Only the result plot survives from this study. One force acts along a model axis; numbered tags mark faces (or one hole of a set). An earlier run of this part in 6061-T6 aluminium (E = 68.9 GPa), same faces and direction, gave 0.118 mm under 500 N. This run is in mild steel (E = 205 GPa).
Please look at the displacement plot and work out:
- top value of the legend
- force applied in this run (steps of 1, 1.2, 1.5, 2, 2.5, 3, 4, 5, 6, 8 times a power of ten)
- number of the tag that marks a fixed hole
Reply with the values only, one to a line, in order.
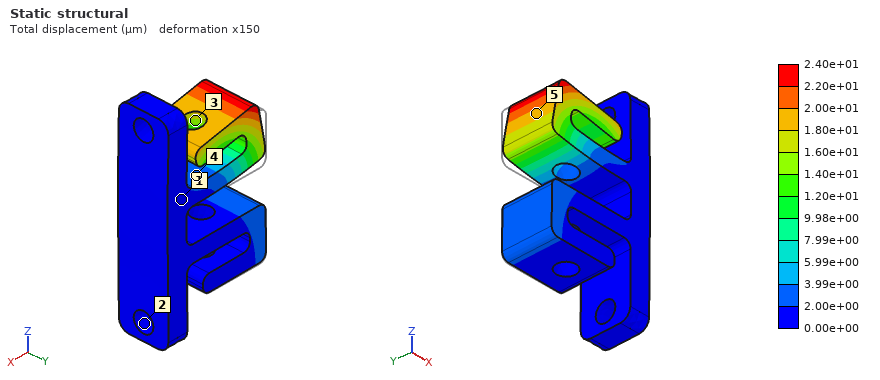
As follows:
2.40e+01 µm
300 N
2
